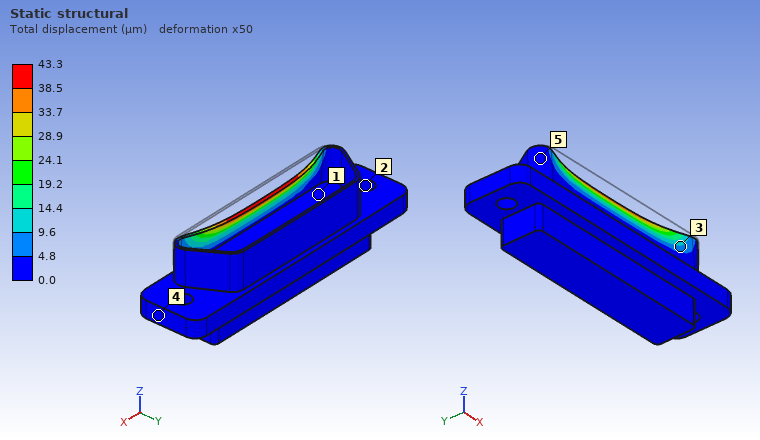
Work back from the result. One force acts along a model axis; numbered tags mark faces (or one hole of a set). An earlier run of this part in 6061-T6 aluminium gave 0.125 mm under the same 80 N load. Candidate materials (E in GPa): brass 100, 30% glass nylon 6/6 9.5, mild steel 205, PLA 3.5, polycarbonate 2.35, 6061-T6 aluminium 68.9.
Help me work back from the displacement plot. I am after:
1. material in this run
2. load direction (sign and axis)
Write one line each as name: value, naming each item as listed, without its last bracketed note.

material in this run: mild steel
load direction: +Y
